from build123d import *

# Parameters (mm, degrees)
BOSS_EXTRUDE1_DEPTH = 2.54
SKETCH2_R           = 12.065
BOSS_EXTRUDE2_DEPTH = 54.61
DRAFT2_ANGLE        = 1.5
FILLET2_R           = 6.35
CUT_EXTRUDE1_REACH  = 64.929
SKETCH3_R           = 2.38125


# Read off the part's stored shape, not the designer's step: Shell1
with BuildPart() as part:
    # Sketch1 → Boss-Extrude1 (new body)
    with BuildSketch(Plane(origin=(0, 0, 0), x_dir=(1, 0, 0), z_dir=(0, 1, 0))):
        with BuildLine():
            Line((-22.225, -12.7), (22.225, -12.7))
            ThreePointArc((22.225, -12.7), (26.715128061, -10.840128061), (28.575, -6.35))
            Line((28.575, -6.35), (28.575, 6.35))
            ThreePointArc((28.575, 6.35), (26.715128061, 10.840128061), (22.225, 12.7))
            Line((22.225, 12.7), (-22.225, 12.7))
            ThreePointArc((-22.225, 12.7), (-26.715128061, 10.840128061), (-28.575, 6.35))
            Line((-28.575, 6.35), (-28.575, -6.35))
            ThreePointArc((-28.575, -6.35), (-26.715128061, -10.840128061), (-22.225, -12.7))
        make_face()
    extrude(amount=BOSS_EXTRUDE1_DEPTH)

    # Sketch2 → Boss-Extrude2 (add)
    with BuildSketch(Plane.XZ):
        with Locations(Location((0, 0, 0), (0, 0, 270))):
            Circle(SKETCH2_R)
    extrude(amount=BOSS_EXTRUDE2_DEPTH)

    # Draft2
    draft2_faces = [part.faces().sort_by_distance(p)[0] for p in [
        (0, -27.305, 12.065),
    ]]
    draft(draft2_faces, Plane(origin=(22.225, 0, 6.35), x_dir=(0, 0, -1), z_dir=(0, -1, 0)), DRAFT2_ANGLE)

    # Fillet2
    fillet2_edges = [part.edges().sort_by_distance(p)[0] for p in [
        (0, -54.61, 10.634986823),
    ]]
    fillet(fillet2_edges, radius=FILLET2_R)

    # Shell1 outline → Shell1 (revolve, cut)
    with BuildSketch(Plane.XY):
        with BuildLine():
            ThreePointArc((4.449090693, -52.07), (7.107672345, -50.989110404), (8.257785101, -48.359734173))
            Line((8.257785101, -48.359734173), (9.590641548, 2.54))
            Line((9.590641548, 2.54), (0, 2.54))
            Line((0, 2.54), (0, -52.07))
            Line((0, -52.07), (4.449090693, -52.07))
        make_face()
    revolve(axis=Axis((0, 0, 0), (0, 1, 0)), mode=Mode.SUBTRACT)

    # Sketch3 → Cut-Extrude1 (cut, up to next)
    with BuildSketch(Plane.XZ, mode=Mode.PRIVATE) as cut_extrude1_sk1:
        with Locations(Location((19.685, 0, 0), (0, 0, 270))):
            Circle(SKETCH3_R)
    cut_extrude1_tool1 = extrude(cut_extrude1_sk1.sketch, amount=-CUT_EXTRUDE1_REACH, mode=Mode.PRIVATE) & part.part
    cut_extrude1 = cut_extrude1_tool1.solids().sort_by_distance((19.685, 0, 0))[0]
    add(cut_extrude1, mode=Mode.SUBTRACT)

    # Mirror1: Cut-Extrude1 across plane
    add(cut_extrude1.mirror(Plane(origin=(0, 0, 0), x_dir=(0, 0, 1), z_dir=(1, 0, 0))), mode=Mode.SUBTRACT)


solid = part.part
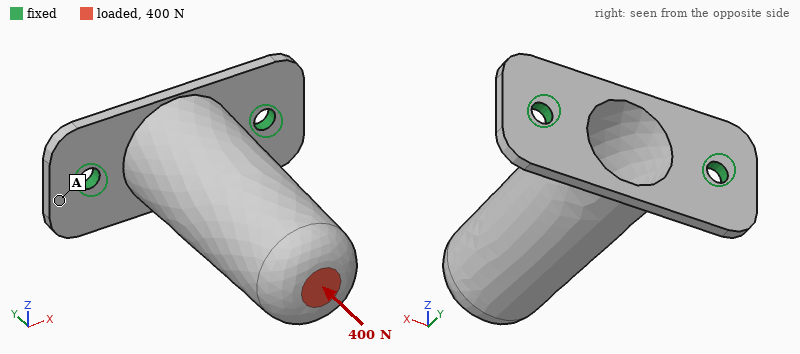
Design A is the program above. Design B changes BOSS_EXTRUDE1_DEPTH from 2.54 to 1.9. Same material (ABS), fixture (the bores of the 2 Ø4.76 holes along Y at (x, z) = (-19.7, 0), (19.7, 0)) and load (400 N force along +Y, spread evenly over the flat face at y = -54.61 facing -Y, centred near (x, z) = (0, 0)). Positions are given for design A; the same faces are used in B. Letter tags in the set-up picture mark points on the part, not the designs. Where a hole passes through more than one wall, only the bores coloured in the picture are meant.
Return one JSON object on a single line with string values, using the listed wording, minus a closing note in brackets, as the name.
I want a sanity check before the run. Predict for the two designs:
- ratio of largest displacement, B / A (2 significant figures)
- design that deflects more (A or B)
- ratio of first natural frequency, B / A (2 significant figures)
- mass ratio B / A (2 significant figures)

{"ratio of largest displacement, B / A": "1.4", "design that deflects more": "B", "ratio of first natural frequency, B / A": "0.72", "mass ratio B / A": "0.94"}
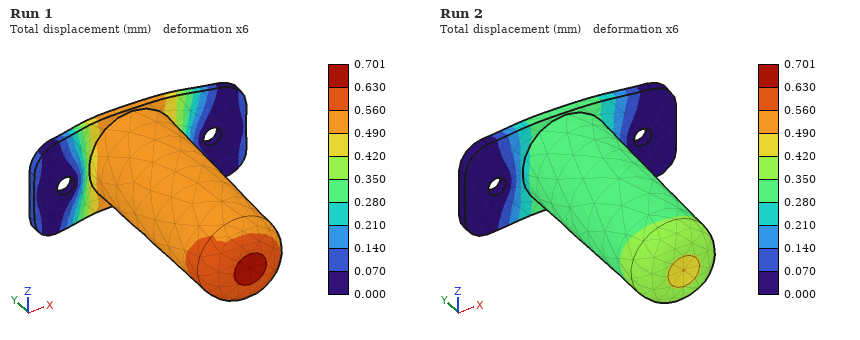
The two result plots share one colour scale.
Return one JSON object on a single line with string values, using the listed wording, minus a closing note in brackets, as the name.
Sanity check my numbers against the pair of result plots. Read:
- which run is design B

{"which run is design B": "Run 1"}
